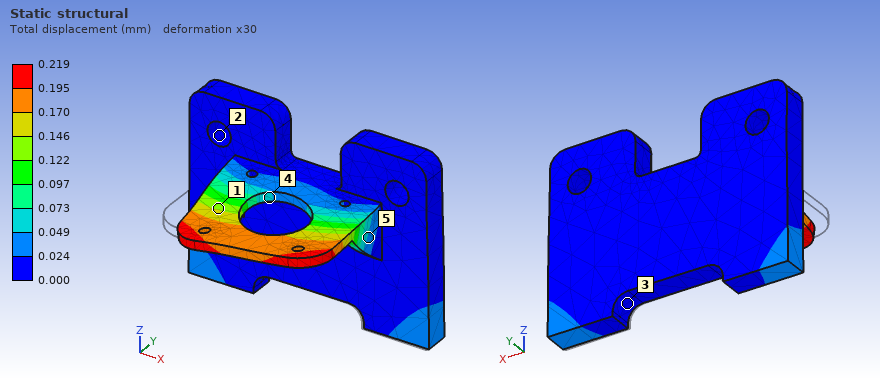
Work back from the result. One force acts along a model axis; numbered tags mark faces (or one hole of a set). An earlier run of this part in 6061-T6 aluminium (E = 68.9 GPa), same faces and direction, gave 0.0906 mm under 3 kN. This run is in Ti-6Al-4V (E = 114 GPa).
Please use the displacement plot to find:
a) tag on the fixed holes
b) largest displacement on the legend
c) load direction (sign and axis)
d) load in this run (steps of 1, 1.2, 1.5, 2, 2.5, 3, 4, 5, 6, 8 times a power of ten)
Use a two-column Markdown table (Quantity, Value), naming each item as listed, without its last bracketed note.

| Quantity | Value |
|---|---|
| tag on the fixed holes | 2 |
| largest displacement on the legend | 0.219 mm |
| load direction | +X |
| load in this run | 12 kN |
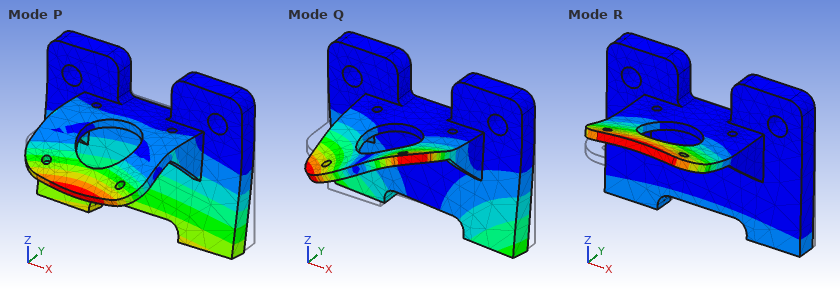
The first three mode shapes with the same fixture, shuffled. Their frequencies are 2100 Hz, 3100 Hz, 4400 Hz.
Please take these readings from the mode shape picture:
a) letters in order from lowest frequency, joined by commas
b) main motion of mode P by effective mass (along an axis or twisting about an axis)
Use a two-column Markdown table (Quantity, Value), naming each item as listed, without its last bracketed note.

| Quantity | Value |
|---|---|
| letters in order from lowest frequency, joined by commas | R, P, Q |
| main motion of mode P by effective mass | along Y |
